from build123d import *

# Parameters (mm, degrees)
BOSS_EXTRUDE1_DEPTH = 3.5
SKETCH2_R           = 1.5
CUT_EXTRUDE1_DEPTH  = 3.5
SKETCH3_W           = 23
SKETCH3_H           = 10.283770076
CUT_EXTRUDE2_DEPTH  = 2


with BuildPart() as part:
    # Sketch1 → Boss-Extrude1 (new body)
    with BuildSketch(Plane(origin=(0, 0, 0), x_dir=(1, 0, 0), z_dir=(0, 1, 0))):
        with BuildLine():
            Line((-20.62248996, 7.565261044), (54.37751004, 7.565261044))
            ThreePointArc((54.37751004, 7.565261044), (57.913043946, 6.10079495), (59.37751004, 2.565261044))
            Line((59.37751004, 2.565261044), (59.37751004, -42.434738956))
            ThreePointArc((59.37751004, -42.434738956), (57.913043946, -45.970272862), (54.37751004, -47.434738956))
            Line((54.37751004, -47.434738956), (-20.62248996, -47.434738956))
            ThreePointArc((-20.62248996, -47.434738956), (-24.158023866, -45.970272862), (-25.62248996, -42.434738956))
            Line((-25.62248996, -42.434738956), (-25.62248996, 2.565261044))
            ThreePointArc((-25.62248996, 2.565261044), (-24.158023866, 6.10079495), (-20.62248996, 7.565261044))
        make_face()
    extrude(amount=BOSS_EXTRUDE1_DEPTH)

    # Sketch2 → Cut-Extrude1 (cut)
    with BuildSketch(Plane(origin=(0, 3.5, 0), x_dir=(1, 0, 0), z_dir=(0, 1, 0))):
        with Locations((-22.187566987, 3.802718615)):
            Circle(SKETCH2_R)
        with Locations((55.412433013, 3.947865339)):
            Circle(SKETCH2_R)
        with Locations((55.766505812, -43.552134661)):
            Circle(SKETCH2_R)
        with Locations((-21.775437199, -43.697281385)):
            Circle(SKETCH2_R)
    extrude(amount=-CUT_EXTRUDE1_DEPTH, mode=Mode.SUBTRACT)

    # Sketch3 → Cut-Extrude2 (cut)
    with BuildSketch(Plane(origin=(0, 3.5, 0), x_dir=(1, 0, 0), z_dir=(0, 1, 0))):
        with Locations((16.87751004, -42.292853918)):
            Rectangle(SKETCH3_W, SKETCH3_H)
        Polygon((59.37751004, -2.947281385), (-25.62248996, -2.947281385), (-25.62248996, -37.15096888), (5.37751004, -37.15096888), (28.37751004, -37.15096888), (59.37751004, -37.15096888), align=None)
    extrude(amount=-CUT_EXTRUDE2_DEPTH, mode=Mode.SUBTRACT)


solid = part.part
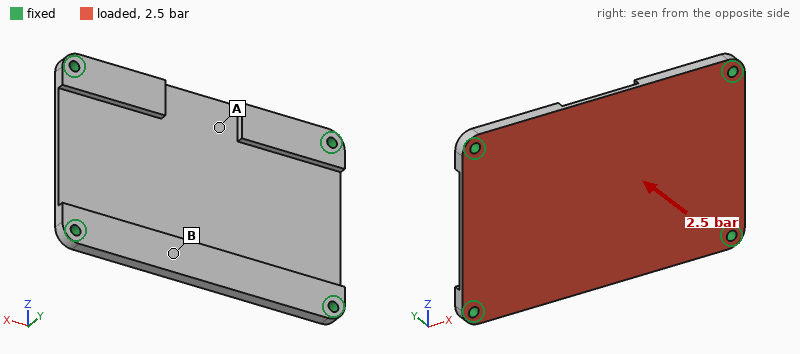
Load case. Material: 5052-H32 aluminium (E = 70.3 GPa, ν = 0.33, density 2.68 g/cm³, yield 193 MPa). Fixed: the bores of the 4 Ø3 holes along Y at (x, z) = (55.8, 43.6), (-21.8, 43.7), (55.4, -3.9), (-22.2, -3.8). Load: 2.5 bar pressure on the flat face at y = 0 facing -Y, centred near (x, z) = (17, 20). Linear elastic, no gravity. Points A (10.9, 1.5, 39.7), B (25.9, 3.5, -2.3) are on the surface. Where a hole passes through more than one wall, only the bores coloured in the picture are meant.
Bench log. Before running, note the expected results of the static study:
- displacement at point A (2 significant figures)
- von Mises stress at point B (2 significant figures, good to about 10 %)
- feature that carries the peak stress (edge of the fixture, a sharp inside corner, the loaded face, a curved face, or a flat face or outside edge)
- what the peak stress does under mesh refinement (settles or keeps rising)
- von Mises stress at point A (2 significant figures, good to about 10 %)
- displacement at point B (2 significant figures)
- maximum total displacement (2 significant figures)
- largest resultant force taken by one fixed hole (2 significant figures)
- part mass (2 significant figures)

0.28 mm
59 MPa
edge of the fixture
keeps rising
26 MPa
0.18 mm
0.37 mm
830 N
27 g
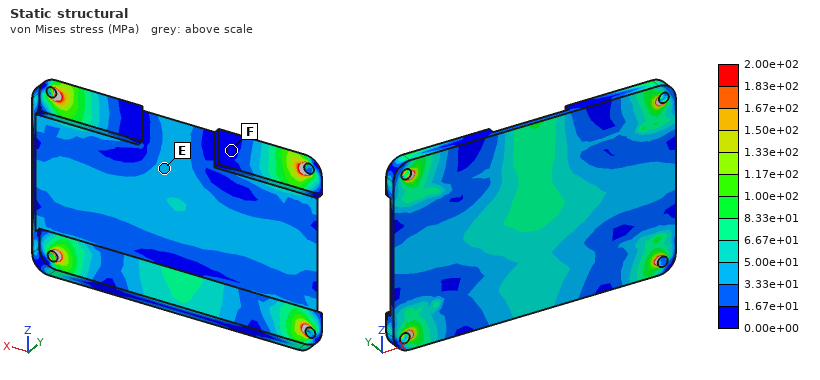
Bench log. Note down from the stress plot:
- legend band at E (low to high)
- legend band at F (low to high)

3.33e+01 to 5.00e+01 MPa
0.00e+00 to 1.67e+01 MPa
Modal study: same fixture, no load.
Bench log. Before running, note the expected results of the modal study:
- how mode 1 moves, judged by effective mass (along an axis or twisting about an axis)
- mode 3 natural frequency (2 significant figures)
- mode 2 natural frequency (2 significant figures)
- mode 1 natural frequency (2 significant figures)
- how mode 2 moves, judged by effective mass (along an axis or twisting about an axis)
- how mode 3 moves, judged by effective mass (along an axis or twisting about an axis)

along Y
4800 Hz
3300 Hz
2400 Hz
twisting about X
twisting about Z
